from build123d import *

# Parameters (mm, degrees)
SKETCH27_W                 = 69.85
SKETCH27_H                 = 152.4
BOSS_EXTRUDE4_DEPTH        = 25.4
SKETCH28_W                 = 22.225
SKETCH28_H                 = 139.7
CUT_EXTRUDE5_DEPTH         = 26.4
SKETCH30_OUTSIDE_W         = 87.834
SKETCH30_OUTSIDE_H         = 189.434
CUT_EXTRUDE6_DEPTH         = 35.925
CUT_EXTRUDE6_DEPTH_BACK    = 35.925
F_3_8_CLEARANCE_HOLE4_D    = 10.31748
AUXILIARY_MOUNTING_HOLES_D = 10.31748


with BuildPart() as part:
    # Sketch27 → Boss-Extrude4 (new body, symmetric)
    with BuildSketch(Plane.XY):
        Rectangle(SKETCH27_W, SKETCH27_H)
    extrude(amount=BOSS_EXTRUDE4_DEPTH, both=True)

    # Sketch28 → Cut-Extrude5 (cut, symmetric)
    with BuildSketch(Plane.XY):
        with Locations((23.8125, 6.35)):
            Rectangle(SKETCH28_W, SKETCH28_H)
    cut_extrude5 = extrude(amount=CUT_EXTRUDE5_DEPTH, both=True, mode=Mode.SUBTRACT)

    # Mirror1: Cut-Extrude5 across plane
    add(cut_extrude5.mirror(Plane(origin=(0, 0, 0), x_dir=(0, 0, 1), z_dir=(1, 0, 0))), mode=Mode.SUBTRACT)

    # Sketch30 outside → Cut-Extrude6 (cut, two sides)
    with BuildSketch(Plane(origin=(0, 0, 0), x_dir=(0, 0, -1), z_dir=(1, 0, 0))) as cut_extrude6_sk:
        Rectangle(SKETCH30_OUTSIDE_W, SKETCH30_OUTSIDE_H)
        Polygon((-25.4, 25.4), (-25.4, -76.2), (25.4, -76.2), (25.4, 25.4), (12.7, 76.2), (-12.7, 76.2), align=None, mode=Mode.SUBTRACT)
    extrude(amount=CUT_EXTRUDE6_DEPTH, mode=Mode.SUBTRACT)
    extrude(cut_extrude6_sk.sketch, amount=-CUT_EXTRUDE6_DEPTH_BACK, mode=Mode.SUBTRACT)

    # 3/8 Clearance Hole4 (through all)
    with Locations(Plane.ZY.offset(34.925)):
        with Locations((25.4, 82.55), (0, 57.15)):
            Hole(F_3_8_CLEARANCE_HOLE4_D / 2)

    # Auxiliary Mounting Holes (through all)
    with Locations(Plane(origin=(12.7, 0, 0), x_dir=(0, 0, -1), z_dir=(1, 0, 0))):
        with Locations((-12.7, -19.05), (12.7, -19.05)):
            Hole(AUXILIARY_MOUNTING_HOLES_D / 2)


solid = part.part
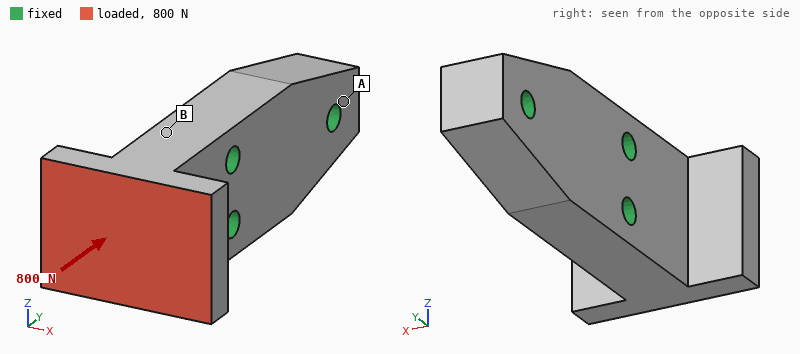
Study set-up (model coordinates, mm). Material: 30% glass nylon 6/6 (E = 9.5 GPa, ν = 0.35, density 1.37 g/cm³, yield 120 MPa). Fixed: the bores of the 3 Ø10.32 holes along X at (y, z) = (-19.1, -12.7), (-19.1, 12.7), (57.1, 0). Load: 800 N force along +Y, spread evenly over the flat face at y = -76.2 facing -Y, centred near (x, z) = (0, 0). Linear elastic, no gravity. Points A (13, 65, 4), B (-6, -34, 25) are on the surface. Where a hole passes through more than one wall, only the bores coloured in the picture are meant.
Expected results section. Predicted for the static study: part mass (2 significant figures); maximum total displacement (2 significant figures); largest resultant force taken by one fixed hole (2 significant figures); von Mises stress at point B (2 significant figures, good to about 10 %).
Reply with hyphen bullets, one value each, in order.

- 280 g
- 15 µm
- 400 N
- 0.45 MPa
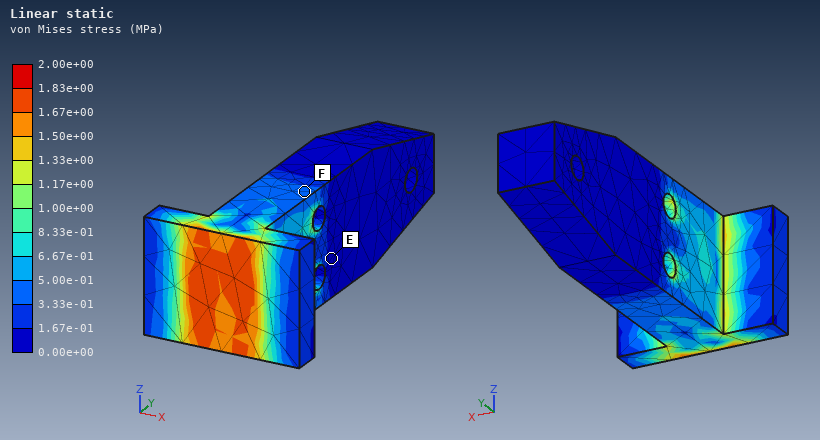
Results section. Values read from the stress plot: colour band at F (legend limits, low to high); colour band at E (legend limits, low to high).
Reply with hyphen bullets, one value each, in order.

- 3.33e-01 to 5.00e-01 MPa
- 0.00e+00 to 1.67e-01 MPa
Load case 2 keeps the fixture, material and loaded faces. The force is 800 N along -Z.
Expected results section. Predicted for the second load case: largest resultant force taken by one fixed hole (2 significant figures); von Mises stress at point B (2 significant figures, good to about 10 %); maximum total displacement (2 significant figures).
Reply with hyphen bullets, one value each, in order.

- 1.3 kN
- 2.7 MPa
- 37 µm
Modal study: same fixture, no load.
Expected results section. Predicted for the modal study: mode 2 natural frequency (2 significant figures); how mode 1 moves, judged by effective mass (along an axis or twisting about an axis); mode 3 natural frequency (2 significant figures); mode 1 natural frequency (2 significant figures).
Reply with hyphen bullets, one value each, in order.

- 3100 Hz
- along X
- 3200 Hz
- 1900 Hz
